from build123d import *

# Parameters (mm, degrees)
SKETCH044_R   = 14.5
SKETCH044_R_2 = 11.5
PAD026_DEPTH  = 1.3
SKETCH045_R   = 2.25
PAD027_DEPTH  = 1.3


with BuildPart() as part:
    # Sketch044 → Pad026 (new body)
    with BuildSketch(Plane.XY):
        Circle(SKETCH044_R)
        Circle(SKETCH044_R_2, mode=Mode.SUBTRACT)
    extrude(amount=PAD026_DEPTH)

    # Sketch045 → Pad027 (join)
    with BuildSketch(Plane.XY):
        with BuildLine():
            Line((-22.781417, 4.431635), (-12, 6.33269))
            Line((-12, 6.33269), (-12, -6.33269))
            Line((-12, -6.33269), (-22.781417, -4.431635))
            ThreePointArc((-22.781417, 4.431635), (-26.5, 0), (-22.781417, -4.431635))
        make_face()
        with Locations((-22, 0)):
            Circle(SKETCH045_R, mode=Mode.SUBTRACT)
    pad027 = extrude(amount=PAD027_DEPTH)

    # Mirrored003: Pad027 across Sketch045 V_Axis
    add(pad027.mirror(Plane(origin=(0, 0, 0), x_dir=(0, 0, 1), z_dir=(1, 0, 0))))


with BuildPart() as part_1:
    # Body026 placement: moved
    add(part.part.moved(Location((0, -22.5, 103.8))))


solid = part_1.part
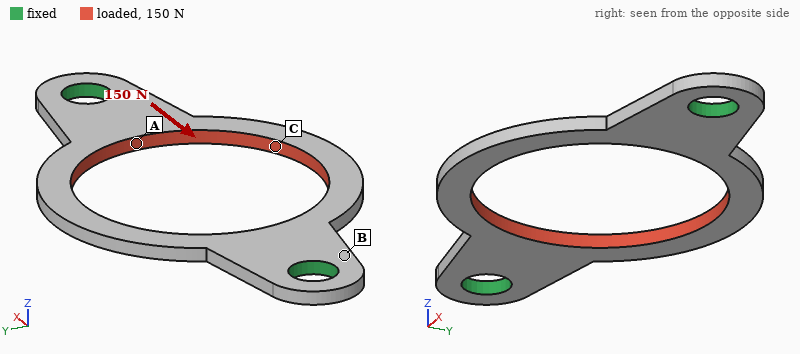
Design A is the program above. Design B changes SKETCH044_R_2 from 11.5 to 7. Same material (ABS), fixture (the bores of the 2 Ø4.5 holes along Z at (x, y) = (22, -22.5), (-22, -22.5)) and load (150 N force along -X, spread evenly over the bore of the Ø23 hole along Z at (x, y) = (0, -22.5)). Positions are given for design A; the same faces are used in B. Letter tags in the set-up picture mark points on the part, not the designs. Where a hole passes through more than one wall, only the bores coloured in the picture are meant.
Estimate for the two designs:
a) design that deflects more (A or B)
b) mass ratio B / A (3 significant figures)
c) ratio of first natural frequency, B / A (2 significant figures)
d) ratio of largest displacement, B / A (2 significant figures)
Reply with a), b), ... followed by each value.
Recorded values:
a) A
b) 1.59
c) 0.92
d) 0.24
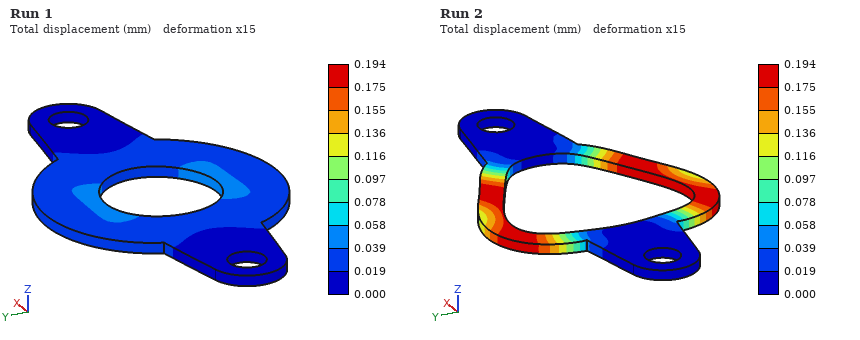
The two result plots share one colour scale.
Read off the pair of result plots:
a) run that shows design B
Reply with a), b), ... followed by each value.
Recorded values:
a) Run 1
